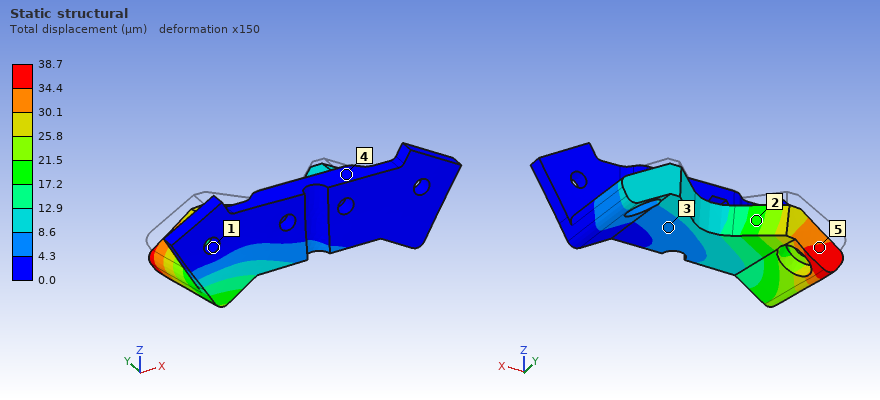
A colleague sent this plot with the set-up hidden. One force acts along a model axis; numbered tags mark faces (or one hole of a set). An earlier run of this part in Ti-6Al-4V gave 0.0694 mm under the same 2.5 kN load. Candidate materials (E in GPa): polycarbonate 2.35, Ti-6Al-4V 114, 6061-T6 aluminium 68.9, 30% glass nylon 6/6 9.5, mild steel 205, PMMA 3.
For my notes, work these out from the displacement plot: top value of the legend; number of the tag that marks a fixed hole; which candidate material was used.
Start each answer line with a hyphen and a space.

- 38.7 µm
- 1
- mild steel
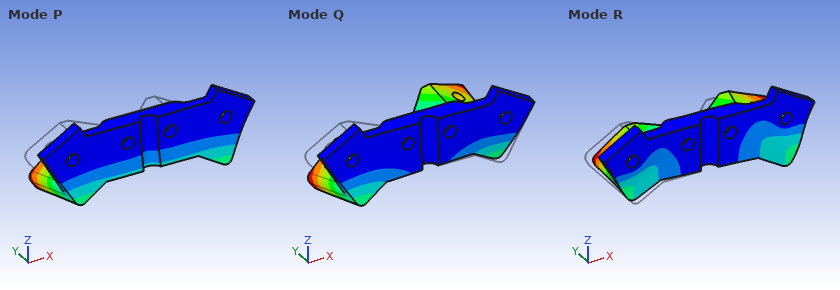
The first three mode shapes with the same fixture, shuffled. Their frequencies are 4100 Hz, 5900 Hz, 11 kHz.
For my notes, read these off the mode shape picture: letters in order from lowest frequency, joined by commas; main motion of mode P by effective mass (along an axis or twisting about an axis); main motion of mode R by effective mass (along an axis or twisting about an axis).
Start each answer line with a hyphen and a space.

- P, Q, R
- along Z
- along X
